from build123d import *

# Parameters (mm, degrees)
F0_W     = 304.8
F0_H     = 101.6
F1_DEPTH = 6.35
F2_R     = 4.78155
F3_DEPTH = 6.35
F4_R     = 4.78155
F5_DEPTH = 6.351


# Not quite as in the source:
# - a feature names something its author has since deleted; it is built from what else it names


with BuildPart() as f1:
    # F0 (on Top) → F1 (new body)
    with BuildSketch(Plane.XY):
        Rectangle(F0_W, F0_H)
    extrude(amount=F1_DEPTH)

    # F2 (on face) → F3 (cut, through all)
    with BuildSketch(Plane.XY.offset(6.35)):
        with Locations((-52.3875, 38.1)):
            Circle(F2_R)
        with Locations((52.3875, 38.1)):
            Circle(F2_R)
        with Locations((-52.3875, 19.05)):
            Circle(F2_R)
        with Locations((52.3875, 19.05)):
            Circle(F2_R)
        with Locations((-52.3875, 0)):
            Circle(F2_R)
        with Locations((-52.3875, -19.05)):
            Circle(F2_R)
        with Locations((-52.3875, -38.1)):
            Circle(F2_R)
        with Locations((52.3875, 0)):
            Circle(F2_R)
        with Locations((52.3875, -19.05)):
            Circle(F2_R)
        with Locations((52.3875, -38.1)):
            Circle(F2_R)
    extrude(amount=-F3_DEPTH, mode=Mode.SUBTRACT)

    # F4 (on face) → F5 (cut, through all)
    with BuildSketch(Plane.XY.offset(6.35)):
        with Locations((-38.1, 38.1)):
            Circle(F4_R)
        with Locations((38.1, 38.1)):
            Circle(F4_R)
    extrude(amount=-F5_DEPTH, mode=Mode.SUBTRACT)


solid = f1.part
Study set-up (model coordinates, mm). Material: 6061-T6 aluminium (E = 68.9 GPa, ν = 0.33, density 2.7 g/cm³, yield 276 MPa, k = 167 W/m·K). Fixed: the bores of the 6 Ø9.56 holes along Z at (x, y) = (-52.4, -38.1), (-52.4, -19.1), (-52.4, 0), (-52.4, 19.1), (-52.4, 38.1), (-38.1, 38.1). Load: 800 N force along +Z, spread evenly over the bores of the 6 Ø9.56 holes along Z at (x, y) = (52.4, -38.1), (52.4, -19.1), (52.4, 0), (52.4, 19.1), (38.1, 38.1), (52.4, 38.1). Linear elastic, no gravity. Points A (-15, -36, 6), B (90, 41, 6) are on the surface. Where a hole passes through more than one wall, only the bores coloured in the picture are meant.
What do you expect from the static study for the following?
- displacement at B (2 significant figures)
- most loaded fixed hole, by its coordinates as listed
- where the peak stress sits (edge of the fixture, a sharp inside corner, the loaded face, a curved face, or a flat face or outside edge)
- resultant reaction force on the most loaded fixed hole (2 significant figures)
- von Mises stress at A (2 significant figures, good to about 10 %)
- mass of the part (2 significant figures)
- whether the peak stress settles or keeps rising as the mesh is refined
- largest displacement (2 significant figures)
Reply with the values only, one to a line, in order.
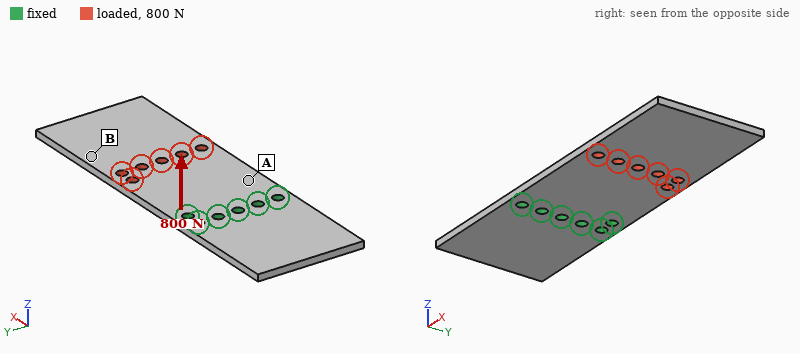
2.2 mm
(-38.1, 38.1)
edge of the fixture
1.1 kN
63 MPa
520 g
keeps rising
3.7 mm
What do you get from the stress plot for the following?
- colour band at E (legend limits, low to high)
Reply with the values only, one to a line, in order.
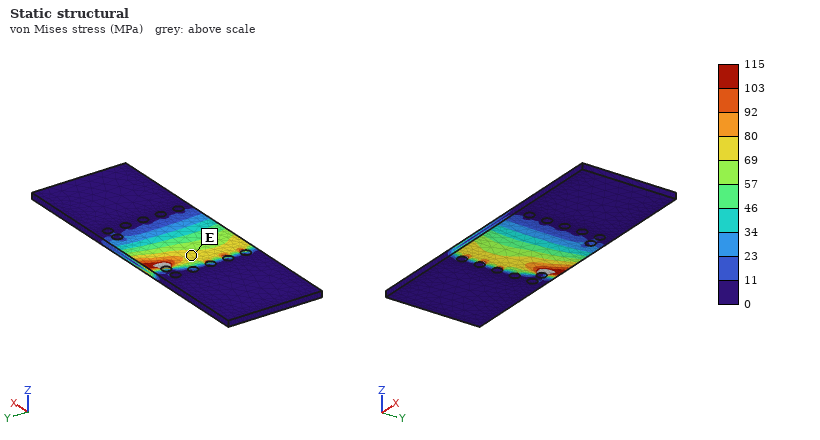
69 to 80 MPa
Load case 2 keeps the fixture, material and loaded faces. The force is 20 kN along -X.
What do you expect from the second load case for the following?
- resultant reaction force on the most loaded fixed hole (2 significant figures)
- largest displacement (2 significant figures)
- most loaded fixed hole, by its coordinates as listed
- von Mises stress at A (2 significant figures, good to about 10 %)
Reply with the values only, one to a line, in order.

6.2 kN
65 µm
(-38.1, 38.1)
23 MPa
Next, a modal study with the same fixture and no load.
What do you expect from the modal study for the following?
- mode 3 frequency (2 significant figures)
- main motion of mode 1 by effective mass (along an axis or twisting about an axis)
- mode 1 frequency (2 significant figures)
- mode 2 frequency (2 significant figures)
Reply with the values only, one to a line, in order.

570 Hz
along Z
140 Hz
550 Hz
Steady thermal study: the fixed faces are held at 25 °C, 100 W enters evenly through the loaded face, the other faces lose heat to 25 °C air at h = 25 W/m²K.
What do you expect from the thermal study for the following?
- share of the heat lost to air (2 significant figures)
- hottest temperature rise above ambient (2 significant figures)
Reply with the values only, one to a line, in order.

41 %
61 K
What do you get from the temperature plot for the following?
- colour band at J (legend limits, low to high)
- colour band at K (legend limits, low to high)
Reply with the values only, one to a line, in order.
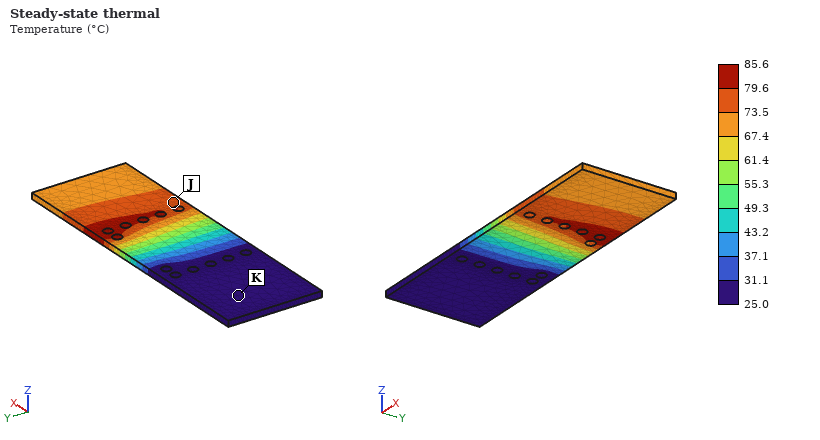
73.5 to 79.6 °C
25.0 to 31.1 °C
